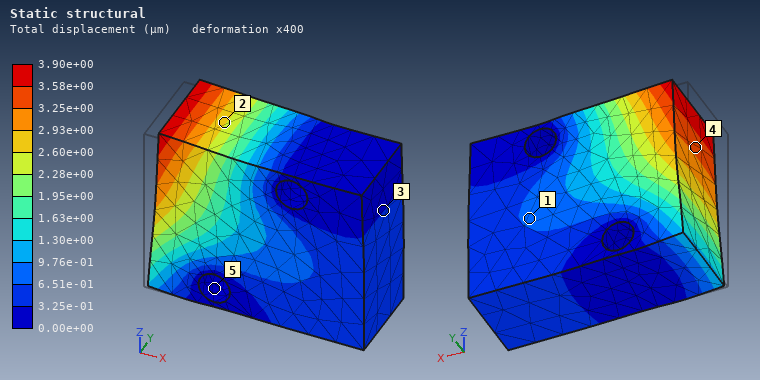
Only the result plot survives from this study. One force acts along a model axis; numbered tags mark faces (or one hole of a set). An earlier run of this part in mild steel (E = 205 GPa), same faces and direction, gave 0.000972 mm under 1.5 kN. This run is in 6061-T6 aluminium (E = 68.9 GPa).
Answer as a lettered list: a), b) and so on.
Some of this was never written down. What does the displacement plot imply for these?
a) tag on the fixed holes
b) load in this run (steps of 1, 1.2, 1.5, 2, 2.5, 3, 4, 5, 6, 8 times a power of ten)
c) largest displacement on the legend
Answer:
a) 5
b) 2 kN
c) 3.90e+00 µm
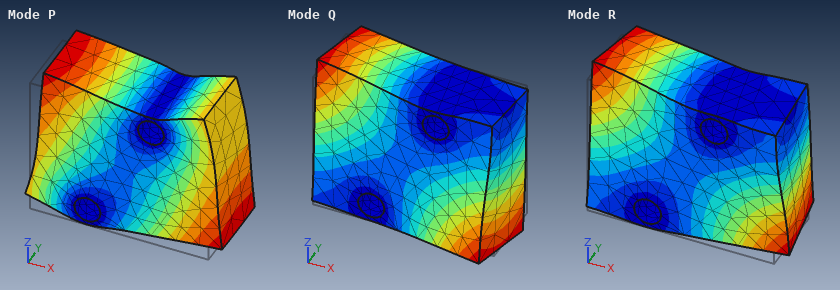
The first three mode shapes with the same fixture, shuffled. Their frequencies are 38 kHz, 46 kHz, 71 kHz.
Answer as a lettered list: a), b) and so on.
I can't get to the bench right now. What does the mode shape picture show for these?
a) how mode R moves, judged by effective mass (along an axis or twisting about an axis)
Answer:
a) along Y
